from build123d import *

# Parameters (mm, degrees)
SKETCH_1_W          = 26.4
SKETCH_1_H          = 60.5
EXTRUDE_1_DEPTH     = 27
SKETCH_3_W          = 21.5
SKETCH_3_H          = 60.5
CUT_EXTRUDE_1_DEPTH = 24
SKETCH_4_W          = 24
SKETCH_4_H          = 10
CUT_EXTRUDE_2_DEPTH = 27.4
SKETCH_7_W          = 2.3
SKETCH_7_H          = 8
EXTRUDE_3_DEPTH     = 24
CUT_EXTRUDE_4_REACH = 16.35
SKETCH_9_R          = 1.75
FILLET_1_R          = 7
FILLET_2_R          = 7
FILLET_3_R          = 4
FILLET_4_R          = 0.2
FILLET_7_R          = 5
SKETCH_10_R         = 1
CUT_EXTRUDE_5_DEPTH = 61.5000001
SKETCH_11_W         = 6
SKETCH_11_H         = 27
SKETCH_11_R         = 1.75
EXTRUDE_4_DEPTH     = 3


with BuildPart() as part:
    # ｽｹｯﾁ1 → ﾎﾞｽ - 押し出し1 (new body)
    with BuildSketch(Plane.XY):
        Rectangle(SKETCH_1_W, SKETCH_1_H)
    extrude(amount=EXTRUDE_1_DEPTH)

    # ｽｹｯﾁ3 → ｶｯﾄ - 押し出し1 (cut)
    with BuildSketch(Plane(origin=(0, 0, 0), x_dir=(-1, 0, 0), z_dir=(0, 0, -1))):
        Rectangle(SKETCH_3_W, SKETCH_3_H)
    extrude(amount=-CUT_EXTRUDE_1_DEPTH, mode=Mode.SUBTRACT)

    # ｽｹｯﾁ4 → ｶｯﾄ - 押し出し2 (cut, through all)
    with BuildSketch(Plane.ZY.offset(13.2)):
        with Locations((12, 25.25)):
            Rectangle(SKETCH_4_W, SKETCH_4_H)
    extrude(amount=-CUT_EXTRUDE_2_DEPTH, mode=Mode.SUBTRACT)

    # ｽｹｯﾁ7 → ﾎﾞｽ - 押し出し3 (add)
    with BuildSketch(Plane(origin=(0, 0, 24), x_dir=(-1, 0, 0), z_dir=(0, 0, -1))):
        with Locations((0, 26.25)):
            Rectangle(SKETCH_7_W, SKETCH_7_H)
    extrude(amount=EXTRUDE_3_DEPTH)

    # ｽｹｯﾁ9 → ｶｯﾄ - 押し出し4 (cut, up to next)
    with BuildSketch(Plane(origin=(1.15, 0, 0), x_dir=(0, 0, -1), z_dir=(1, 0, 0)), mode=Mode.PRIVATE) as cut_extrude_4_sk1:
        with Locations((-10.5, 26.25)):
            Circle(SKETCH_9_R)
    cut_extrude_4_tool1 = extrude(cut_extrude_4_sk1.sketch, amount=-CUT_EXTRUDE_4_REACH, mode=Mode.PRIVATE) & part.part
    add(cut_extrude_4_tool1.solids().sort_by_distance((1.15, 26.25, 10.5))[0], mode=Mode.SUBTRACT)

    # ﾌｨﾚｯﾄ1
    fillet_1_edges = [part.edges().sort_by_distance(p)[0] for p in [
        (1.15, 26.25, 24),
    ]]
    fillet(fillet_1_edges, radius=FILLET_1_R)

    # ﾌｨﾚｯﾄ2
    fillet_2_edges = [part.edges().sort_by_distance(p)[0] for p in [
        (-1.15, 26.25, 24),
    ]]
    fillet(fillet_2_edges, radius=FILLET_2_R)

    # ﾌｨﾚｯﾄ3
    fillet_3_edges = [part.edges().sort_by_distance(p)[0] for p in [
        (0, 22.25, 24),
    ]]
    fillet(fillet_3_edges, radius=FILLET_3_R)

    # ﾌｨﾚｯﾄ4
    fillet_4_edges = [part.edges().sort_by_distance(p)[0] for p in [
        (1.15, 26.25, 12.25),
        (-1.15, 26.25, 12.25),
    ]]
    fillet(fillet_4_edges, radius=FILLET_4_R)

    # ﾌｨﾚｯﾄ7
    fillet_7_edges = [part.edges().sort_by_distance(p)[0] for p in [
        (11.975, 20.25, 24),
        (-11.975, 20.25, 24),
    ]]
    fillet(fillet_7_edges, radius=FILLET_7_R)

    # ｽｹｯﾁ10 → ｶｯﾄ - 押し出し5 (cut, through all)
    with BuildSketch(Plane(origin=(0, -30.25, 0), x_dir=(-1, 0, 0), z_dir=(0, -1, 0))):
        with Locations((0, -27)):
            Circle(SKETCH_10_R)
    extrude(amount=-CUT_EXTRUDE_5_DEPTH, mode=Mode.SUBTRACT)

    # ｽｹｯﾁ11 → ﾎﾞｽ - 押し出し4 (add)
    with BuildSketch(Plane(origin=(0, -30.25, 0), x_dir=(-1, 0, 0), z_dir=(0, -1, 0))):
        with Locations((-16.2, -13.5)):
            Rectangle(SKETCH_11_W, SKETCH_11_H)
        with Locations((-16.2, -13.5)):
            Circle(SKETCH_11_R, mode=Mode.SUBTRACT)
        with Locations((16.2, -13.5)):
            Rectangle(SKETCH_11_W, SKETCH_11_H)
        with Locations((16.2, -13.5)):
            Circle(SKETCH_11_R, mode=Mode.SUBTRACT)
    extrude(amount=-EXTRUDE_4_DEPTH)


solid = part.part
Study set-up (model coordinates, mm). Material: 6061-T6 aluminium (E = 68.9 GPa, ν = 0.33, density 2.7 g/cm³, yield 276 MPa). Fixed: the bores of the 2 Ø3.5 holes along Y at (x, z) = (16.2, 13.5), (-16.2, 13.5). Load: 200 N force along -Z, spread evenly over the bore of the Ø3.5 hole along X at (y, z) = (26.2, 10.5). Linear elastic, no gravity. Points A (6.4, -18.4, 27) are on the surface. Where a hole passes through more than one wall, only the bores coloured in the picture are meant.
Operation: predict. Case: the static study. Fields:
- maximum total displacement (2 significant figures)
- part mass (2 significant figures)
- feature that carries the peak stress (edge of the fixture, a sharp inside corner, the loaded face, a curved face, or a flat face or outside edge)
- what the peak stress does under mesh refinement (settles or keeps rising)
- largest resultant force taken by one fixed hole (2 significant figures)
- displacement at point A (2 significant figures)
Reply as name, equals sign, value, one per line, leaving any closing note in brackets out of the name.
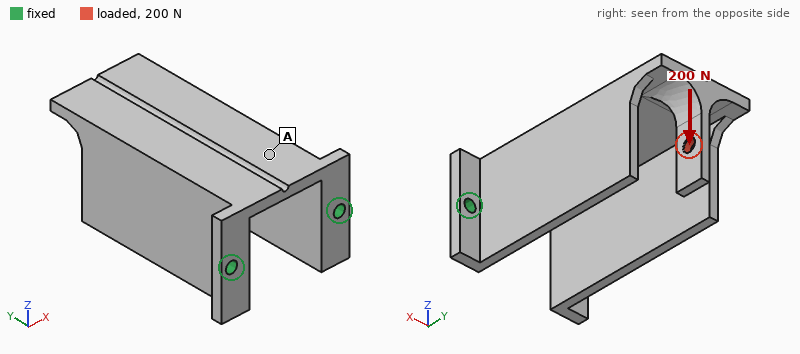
maximum total displacement = 0.36 mm
part mass = 33 g
feature that carries the peak stress = edge of the fixture
what the peak stress does under mesh refinement = keeps rising
largest resultant force taken by one fixed hole = 100 N
displacement at point A = 0.086 mm
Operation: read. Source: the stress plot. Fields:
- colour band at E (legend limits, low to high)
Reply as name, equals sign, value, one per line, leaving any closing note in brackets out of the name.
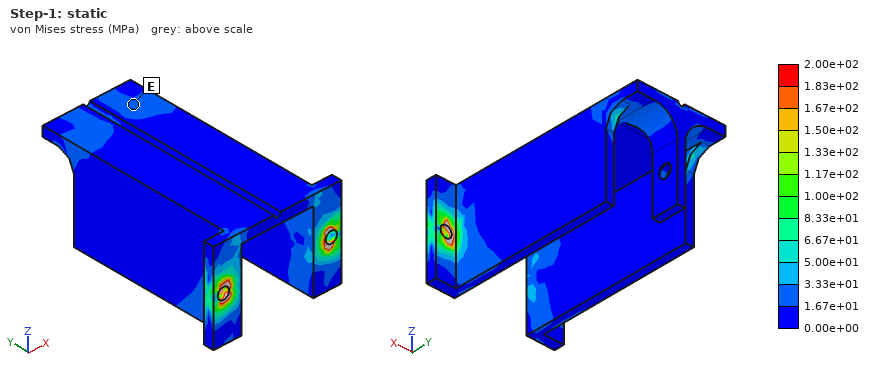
colour band at E = 1.67e+01 to 3.33e+01 MPa
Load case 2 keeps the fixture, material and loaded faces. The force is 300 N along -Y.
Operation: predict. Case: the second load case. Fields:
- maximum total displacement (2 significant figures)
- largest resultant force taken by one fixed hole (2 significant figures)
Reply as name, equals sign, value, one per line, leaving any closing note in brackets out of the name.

maximum total displacement = 0.25 mm
largest resultant force taken by one fixed hole = 150 N
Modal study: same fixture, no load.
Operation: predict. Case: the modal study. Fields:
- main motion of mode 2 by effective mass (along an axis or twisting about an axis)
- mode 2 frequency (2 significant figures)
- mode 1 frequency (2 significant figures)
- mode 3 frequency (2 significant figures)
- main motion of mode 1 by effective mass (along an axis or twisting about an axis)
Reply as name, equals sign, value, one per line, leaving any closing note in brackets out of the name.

main motion of mode 2 by effective mass = along X
mode 2 frequency = 1400 Hz
mode 1 frequency = 1200 Hz
mode 3 frequency = 3300 Hz
main motion of mode 1 by effective mass = along Z
